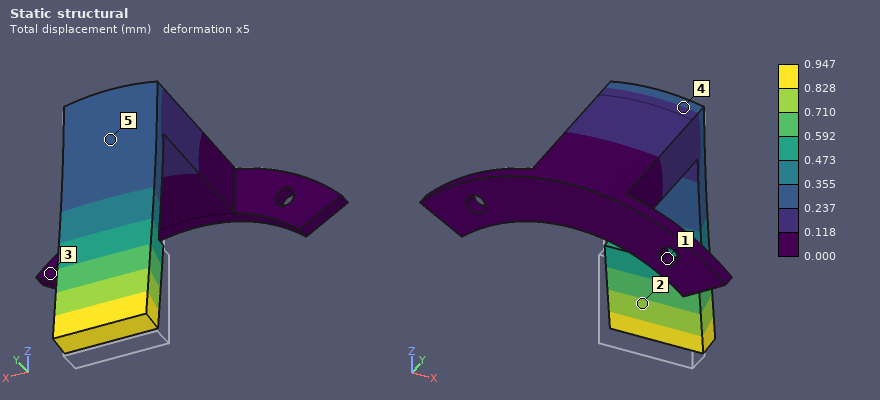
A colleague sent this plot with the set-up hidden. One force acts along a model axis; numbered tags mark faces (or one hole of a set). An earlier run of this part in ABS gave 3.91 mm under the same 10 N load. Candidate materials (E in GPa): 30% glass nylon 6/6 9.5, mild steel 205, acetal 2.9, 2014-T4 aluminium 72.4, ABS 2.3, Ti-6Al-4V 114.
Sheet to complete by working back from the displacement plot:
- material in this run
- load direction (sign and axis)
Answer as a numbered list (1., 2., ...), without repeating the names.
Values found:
1. 30% glass nylon 6/6
2. +Y
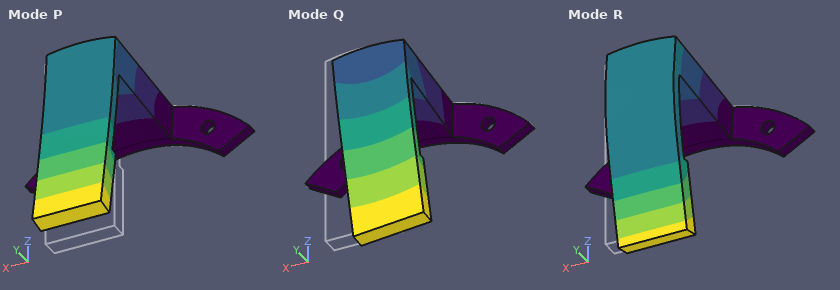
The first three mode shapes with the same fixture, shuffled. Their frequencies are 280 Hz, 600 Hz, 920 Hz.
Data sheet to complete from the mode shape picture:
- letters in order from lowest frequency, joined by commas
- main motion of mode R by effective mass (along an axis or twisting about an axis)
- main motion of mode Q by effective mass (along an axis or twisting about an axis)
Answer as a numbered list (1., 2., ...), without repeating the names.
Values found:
1. P, R, Q
2. along Z
3. along X
